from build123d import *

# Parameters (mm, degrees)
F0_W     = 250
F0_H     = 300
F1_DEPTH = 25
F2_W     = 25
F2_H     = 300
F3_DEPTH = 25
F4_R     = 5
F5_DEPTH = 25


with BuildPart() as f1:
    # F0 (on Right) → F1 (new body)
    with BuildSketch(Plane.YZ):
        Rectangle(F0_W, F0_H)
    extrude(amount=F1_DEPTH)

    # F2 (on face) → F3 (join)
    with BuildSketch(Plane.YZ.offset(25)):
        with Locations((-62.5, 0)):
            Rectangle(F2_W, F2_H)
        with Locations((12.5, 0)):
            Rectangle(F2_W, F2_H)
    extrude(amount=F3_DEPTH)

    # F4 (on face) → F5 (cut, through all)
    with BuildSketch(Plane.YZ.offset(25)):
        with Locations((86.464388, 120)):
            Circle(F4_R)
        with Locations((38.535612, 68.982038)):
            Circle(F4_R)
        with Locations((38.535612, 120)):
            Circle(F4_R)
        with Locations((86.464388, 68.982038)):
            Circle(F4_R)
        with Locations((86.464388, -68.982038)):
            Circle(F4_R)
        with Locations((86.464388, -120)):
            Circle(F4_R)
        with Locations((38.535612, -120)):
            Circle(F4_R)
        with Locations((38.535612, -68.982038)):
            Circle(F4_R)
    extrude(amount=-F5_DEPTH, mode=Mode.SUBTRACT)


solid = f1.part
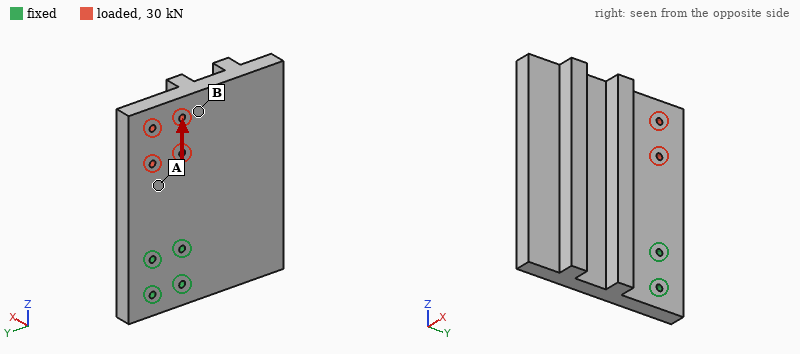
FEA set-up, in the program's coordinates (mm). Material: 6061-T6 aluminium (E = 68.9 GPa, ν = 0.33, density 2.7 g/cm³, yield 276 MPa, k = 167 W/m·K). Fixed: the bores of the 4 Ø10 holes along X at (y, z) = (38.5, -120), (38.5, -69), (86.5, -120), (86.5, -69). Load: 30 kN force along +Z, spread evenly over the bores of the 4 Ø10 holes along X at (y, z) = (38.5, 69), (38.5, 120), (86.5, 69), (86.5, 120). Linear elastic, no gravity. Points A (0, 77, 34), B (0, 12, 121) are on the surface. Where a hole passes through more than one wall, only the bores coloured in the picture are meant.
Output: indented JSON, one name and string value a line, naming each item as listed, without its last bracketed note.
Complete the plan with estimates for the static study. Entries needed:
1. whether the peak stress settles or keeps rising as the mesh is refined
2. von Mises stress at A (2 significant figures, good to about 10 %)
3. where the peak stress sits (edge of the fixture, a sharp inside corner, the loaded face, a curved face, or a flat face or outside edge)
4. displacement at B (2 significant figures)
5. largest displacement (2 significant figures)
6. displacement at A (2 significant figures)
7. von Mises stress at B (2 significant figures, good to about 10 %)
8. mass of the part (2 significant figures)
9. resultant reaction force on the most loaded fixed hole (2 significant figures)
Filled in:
{
  "whether the peak stress settles or keeps rising as the mesh is refined": "keeps rising",
  "von Mises stress at A": "12 MPa",
  "where the peak stress sits": "edge of the fixture",
  "displacement at B": "33 µm",
  "largest displacement": "44 µm",
  "displacement at A": "20 µm",
  "von Mises stress at B": "3.8 MPa",
  "mass of the part": "6.0 kg",
  "resultant reaction force on the most loaded fixed hole": "12 kN"
}
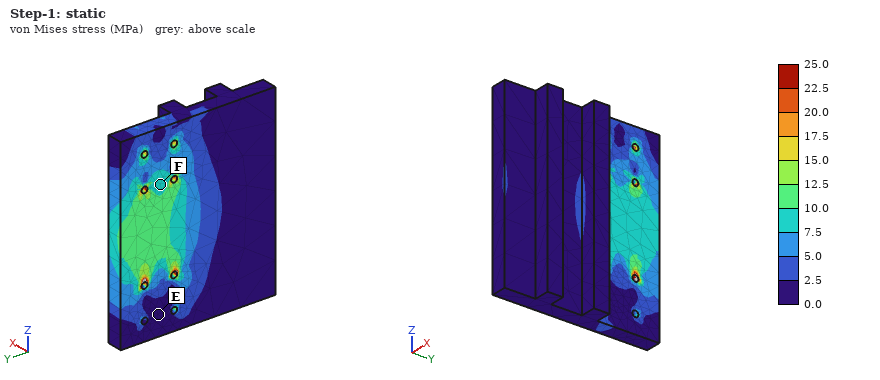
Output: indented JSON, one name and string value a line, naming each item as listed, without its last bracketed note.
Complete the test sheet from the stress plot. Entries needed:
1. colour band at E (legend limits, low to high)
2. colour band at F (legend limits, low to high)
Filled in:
{
  "colour band at E": "0.0 to 2.5 MPa",
  "colour band at F": "7.5 to 10.0 MPa"
}
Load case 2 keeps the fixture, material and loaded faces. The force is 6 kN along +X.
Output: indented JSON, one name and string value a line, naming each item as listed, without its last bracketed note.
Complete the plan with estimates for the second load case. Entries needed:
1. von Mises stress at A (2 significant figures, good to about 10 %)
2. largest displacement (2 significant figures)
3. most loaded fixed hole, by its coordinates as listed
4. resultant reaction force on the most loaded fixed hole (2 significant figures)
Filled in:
{
  "von Mises stress at A": "11 MPa",
  "largest displacement": "0.53 mm",
  "most loaded fixed hole, by its coordinates as listed": "(38.5, -69)",
  "resultant reaction force on the most loaded fixed hole": "12 kN"
}
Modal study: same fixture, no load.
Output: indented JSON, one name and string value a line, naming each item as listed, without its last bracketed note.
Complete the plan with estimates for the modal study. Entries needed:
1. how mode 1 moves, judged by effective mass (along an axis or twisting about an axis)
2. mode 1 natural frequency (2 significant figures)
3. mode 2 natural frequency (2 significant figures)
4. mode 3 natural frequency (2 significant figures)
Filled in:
{
  "how mode 1 moves, judged by effective mass": "along X",
  "mode 1 natural frequency": "370 Hz",
  "mode 2 natural frequency": "630 Hz",
  "mode 3 natural frequency": "1000 Hz"
}
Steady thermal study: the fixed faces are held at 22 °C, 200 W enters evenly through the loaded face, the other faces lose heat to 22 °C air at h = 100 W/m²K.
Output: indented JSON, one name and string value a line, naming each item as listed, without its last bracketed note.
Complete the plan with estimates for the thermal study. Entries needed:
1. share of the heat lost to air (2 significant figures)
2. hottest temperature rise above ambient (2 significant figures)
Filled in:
{
  "share of the heat lost to air": "70 %",
  "hottest temperature rise above ambient": "24 K"
}
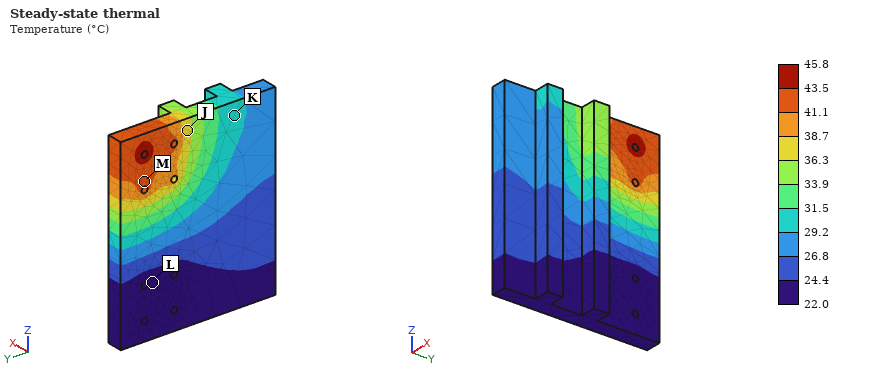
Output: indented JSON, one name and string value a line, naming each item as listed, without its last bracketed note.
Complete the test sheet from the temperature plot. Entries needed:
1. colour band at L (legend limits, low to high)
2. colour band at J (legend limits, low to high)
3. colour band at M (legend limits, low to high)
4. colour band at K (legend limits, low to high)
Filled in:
{
  "colour band at L": "22.0 to 24.4 °C",
  "colour band at J": "36.3 to 38.7 °C",
  "colour band at M": "41.1 to 43.5 °C",
  "colour band at K": "29.2 to 31.5 °C"
}
